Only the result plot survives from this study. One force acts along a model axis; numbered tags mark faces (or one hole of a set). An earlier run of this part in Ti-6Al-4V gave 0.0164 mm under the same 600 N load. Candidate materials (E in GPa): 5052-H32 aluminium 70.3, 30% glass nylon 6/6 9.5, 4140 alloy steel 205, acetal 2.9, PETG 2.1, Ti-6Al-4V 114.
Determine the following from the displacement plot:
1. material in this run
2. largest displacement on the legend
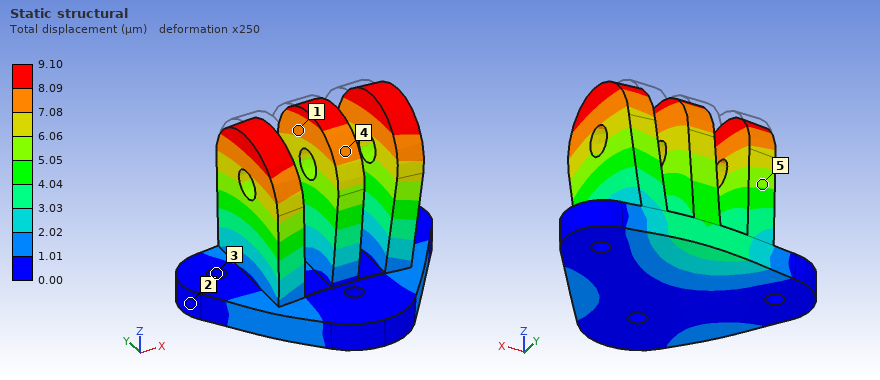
4140 alloy steel
9.10 µm
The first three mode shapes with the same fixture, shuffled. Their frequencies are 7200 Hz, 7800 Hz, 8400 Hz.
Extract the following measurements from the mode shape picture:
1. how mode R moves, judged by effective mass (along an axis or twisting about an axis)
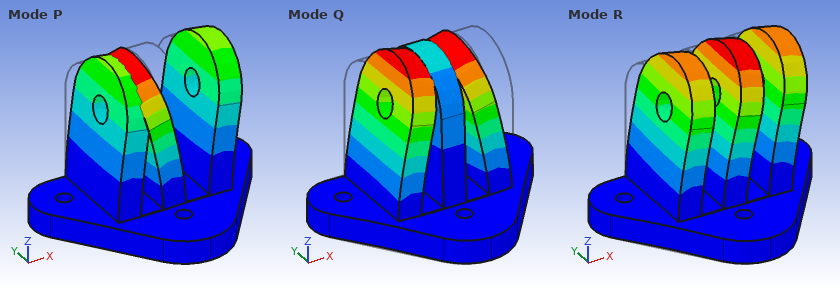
along X
